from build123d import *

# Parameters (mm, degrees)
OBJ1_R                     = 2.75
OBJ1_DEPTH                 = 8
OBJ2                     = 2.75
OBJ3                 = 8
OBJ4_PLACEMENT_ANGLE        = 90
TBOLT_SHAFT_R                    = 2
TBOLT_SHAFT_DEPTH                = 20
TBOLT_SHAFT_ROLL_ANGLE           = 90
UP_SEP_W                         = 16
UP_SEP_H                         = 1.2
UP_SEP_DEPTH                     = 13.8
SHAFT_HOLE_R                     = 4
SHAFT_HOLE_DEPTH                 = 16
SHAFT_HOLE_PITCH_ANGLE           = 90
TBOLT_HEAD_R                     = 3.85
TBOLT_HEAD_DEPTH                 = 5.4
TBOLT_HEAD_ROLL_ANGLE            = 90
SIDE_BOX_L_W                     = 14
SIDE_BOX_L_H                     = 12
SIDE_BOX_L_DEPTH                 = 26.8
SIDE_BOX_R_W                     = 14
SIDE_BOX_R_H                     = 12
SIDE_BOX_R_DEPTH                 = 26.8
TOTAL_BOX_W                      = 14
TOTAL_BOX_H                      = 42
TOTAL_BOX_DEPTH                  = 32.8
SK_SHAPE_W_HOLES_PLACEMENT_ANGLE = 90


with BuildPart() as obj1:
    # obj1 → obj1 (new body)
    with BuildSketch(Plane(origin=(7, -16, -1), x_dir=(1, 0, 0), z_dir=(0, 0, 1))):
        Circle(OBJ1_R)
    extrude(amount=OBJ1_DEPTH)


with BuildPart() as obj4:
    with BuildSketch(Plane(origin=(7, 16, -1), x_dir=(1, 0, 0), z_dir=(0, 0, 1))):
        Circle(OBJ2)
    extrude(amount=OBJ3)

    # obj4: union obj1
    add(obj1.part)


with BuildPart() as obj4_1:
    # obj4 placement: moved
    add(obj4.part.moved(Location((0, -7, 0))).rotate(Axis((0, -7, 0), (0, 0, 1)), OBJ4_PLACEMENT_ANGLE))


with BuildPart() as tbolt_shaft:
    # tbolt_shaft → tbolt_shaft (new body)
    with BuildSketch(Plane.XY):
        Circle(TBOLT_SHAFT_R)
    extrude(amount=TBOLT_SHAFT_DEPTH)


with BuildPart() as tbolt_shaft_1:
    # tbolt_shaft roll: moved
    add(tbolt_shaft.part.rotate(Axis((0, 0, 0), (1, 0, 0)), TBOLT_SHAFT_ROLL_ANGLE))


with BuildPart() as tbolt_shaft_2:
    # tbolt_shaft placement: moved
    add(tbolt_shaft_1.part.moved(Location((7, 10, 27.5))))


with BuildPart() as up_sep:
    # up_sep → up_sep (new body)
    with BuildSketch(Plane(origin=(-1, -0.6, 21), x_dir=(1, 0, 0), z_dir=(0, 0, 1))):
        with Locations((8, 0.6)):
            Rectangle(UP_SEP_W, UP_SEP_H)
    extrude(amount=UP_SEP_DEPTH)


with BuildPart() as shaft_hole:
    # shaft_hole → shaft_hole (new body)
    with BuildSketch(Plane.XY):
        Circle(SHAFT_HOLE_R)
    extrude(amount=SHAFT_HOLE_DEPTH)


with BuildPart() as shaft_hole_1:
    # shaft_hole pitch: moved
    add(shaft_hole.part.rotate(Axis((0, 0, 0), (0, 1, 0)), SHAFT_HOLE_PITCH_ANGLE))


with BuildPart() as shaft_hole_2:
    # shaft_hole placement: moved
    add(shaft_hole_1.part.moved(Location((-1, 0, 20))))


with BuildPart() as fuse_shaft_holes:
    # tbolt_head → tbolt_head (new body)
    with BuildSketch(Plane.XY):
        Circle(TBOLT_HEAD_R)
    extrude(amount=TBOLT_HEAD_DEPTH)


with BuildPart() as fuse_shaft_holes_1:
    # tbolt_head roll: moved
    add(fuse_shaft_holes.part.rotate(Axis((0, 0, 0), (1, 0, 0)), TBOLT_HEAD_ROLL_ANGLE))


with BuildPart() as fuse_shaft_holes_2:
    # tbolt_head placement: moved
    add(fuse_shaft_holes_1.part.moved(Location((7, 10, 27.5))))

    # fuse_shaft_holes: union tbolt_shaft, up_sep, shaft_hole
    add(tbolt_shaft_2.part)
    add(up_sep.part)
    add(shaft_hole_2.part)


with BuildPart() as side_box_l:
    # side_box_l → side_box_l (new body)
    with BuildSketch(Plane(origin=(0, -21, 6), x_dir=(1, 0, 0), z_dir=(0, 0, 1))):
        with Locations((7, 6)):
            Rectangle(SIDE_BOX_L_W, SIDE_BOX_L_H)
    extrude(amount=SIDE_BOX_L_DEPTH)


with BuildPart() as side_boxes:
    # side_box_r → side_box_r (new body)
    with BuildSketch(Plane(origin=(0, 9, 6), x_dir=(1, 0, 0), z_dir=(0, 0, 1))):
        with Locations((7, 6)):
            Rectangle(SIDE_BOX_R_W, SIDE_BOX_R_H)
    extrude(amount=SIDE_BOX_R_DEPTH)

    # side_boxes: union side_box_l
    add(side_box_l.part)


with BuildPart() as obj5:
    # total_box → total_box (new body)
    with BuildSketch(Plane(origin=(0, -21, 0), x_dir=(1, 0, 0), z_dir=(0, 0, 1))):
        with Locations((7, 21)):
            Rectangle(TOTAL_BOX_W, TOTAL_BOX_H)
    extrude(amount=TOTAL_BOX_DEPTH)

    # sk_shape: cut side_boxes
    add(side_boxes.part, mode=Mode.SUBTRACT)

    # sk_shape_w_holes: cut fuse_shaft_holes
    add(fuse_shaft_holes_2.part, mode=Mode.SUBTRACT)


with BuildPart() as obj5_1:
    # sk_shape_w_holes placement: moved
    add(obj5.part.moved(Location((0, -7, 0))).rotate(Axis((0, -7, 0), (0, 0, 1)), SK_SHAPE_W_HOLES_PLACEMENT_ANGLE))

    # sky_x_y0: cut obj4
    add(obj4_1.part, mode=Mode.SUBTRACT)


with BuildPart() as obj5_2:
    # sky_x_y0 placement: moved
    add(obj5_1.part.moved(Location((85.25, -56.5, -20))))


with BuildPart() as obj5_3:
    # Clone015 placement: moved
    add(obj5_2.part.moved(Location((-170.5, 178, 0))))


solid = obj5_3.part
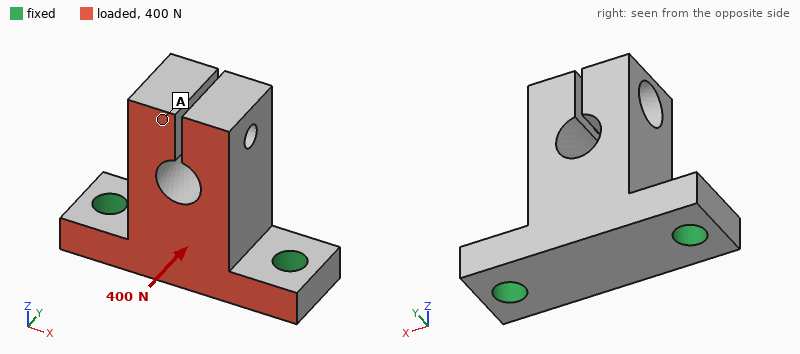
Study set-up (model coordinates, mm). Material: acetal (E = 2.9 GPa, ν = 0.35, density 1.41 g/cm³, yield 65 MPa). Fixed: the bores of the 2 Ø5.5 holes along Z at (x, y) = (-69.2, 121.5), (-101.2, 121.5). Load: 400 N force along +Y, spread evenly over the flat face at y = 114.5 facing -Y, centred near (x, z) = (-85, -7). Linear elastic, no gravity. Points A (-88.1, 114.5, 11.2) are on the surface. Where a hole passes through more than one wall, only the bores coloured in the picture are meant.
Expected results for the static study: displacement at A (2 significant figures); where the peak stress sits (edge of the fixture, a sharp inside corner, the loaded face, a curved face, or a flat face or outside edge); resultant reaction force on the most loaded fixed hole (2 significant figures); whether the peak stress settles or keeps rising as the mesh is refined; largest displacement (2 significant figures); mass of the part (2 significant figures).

0.55 mm
edge of the fixture
200 N
keeps rising
0.58 mm
12 g
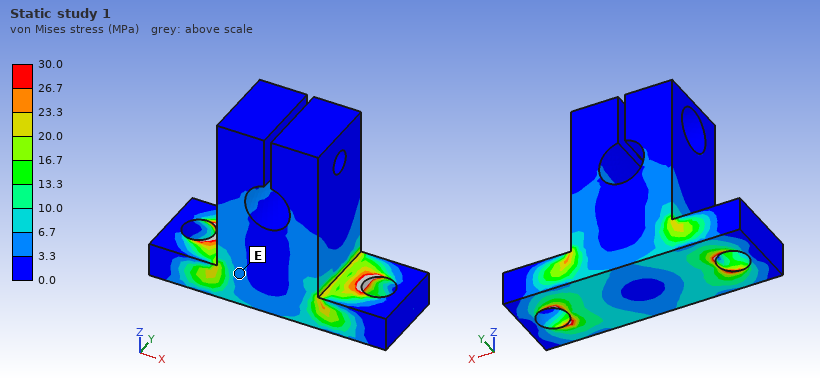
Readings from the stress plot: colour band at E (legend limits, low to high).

3.3 to 6.7 MPa
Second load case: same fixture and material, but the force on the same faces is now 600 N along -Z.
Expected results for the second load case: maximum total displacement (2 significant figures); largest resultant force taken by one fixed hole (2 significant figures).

0.50 mm
310 N
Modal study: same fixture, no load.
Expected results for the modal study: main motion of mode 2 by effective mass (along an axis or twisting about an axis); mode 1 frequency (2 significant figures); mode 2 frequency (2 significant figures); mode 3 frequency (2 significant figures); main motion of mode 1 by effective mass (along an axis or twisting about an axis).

along X
1500 Hz
2400 Hz
2900 Hz
along Y
